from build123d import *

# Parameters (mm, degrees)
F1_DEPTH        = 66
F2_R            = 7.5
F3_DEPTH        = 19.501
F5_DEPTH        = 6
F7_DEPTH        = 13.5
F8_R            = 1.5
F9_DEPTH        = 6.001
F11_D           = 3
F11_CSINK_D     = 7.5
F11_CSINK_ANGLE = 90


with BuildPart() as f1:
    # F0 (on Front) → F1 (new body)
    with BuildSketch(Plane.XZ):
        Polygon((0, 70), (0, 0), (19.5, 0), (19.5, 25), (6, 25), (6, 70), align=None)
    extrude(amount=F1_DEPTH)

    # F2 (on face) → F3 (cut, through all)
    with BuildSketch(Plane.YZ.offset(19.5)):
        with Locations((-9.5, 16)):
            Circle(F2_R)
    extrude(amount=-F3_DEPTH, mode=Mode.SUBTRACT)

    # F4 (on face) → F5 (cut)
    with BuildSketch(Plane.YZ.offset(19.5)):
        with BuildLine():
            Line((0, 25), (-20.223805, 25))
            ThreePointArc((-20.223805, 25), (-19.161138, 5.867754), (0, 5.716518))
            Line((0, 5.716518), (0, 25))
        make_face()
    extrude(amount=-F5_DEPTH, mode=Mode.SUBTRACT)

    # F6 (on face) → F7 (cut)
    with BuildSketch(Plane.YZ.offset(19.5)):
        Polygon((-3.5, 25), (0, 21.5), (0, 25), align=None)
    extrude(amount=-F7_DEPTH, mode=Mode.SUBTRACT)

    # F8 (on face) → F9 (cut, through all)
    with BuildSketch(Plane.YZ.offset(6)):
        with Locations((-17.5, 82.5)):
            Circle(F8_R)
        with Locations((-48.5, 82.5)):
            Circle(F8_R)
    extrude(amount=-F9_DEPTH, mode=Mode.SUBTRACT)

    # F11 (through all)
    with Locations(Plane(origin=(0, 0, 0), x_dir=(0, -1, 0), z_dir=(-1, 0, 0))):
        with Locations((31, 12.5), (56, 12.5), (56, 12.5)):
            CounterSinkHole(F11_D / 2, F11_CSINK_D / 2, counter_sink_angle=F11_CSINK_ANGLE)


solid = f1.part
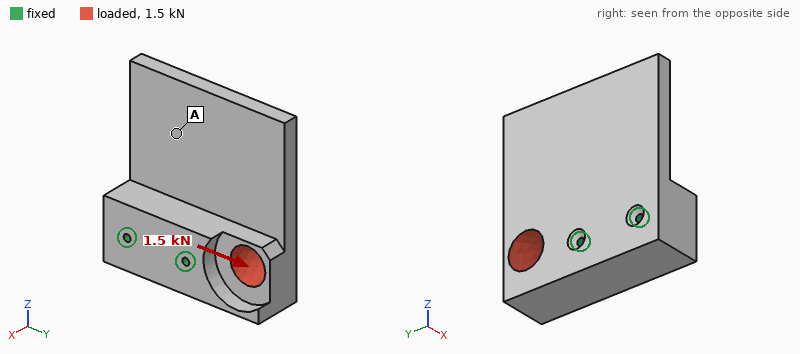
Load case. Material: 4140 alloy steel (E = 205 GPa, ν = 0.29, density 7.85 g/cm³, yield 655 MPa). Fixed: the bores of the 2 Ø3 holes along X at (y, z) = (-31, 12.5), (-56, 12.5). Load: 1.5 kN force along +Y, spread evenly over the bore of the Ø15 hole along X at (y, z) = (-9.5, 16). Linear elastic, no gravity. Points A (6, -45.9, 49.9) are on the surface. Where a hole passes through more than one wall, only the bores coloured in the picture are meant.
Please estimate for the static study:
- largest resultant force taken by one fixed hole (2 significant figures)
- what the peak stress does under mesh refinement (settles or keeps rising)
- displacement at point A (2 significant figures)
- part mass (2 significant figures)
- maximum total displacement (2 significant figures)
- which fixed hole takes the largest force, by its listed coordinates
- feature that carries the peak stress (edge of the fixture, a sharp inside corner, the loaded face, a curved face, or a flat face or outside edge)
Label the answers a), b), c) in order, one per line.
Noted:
a) 1.1 kN
b) keeps rising
c) 0.66 µm
d) 350 g
e) 2.4 µm
f) (-31, 12.5)
g) edge of the fixture
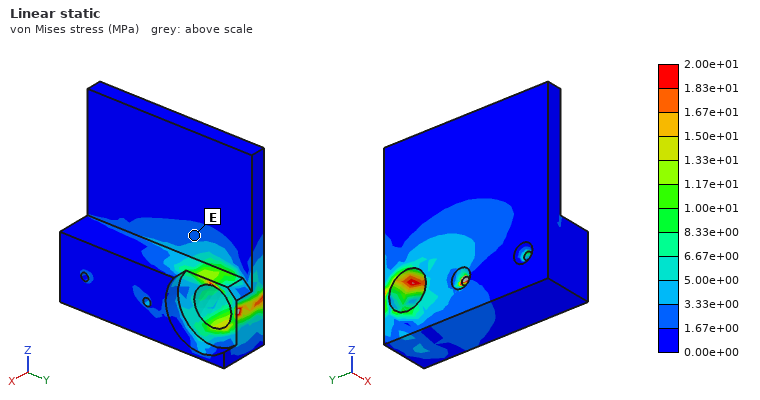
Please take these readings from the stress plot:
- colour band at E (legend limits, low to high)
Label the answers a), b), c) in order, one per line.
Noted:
a) 1.67e+00 to 3.33e+00 MPa
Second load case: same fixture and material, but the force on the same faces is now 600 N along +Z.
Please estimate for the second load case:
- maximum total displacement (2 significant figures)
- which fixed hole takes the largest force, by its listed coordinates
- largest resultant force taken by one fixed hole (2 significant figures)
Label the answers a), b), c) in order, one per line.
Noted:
a) 2.4 µm
b) (-31, 12.5)
c) 1.1 kN
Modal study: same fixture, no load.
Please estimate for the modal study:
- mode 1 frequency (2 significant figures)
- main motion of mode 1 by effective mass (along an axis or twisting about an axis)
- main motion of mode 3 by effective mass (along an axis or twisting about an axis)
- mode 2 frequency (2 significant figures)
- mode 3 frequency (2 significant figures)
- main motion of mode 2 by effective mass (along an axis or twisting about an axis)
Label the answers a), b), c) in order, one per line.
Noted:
a) 2000 Hz
b) along X
c) along Y
d) 3700 Hz
e) 6600 Hz
f) twisting about Z
